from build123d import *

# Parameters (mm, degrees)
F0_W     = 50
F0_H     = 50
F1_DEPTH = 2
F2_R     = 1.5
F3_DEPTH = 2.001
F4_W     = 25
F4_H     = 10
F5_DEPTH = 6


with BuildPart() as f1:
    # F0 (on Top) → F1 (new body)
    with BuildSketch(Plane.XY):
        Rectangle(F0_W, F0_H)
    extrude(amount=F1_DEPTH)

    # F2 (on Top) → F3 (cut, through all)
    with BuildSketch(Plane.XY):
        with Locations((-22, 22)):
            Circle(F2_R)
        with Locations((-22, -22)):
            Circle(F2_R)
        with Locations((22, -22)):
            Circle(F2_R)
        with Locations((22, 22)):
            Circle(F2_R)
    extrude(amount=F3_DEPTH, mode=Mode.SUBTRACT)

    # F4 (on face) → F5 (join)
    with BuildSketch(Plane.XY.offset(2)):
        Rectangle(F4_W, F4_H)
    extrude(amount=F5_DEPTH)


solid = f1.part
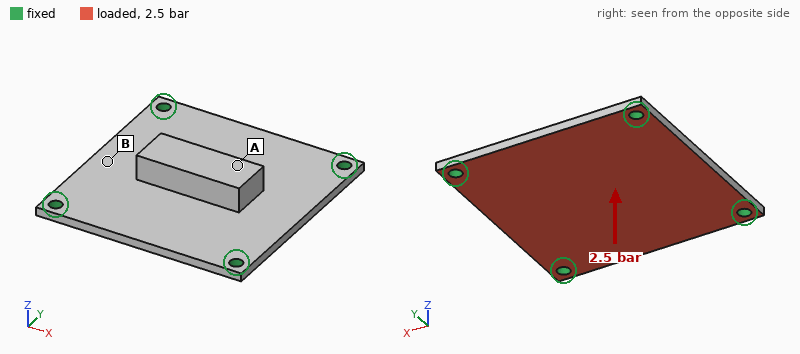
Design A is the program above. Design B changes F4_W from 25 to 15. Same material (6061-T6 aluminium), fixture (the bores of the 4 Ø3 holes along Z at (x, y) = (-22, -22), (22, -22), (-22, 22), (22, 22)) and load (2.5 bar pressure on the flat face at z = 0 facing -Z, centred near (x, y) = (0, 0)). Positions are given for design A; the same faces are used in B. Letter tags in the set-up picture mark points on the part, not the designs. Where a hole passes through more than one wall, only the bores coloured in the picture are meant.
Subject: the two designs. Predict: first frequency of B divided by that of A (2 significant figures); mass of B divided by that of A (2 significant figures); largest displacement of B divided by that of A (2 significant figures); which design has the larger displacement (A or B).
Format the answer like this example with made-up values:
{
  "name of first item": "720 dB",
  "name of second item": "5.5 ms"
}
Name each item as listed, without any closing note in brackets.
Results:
{
  "first frequency of B divided by that of A": "1.0",
  "mass of B divided by that of A": "0.91",
  "largest displacement of B divided by that of A": "1.2",
  "which design has the larger displacement": "B"
}
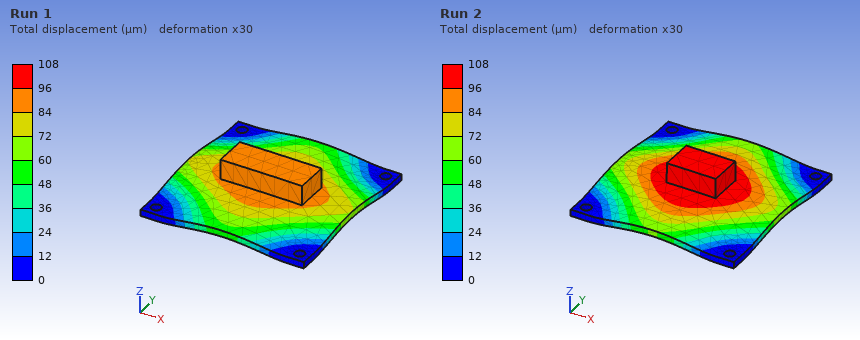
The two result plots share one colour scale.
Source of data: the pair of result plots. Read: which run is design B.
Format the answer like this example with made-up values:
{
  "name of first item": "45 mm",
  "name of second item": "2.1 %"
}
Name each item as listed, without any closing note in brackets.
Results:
{
  "which run is design B": "Run 2"
}
